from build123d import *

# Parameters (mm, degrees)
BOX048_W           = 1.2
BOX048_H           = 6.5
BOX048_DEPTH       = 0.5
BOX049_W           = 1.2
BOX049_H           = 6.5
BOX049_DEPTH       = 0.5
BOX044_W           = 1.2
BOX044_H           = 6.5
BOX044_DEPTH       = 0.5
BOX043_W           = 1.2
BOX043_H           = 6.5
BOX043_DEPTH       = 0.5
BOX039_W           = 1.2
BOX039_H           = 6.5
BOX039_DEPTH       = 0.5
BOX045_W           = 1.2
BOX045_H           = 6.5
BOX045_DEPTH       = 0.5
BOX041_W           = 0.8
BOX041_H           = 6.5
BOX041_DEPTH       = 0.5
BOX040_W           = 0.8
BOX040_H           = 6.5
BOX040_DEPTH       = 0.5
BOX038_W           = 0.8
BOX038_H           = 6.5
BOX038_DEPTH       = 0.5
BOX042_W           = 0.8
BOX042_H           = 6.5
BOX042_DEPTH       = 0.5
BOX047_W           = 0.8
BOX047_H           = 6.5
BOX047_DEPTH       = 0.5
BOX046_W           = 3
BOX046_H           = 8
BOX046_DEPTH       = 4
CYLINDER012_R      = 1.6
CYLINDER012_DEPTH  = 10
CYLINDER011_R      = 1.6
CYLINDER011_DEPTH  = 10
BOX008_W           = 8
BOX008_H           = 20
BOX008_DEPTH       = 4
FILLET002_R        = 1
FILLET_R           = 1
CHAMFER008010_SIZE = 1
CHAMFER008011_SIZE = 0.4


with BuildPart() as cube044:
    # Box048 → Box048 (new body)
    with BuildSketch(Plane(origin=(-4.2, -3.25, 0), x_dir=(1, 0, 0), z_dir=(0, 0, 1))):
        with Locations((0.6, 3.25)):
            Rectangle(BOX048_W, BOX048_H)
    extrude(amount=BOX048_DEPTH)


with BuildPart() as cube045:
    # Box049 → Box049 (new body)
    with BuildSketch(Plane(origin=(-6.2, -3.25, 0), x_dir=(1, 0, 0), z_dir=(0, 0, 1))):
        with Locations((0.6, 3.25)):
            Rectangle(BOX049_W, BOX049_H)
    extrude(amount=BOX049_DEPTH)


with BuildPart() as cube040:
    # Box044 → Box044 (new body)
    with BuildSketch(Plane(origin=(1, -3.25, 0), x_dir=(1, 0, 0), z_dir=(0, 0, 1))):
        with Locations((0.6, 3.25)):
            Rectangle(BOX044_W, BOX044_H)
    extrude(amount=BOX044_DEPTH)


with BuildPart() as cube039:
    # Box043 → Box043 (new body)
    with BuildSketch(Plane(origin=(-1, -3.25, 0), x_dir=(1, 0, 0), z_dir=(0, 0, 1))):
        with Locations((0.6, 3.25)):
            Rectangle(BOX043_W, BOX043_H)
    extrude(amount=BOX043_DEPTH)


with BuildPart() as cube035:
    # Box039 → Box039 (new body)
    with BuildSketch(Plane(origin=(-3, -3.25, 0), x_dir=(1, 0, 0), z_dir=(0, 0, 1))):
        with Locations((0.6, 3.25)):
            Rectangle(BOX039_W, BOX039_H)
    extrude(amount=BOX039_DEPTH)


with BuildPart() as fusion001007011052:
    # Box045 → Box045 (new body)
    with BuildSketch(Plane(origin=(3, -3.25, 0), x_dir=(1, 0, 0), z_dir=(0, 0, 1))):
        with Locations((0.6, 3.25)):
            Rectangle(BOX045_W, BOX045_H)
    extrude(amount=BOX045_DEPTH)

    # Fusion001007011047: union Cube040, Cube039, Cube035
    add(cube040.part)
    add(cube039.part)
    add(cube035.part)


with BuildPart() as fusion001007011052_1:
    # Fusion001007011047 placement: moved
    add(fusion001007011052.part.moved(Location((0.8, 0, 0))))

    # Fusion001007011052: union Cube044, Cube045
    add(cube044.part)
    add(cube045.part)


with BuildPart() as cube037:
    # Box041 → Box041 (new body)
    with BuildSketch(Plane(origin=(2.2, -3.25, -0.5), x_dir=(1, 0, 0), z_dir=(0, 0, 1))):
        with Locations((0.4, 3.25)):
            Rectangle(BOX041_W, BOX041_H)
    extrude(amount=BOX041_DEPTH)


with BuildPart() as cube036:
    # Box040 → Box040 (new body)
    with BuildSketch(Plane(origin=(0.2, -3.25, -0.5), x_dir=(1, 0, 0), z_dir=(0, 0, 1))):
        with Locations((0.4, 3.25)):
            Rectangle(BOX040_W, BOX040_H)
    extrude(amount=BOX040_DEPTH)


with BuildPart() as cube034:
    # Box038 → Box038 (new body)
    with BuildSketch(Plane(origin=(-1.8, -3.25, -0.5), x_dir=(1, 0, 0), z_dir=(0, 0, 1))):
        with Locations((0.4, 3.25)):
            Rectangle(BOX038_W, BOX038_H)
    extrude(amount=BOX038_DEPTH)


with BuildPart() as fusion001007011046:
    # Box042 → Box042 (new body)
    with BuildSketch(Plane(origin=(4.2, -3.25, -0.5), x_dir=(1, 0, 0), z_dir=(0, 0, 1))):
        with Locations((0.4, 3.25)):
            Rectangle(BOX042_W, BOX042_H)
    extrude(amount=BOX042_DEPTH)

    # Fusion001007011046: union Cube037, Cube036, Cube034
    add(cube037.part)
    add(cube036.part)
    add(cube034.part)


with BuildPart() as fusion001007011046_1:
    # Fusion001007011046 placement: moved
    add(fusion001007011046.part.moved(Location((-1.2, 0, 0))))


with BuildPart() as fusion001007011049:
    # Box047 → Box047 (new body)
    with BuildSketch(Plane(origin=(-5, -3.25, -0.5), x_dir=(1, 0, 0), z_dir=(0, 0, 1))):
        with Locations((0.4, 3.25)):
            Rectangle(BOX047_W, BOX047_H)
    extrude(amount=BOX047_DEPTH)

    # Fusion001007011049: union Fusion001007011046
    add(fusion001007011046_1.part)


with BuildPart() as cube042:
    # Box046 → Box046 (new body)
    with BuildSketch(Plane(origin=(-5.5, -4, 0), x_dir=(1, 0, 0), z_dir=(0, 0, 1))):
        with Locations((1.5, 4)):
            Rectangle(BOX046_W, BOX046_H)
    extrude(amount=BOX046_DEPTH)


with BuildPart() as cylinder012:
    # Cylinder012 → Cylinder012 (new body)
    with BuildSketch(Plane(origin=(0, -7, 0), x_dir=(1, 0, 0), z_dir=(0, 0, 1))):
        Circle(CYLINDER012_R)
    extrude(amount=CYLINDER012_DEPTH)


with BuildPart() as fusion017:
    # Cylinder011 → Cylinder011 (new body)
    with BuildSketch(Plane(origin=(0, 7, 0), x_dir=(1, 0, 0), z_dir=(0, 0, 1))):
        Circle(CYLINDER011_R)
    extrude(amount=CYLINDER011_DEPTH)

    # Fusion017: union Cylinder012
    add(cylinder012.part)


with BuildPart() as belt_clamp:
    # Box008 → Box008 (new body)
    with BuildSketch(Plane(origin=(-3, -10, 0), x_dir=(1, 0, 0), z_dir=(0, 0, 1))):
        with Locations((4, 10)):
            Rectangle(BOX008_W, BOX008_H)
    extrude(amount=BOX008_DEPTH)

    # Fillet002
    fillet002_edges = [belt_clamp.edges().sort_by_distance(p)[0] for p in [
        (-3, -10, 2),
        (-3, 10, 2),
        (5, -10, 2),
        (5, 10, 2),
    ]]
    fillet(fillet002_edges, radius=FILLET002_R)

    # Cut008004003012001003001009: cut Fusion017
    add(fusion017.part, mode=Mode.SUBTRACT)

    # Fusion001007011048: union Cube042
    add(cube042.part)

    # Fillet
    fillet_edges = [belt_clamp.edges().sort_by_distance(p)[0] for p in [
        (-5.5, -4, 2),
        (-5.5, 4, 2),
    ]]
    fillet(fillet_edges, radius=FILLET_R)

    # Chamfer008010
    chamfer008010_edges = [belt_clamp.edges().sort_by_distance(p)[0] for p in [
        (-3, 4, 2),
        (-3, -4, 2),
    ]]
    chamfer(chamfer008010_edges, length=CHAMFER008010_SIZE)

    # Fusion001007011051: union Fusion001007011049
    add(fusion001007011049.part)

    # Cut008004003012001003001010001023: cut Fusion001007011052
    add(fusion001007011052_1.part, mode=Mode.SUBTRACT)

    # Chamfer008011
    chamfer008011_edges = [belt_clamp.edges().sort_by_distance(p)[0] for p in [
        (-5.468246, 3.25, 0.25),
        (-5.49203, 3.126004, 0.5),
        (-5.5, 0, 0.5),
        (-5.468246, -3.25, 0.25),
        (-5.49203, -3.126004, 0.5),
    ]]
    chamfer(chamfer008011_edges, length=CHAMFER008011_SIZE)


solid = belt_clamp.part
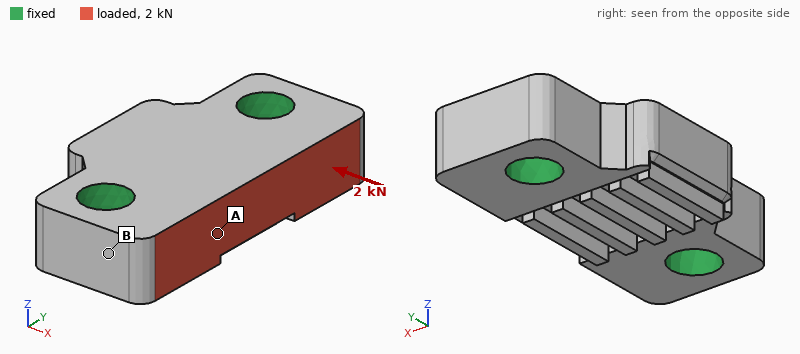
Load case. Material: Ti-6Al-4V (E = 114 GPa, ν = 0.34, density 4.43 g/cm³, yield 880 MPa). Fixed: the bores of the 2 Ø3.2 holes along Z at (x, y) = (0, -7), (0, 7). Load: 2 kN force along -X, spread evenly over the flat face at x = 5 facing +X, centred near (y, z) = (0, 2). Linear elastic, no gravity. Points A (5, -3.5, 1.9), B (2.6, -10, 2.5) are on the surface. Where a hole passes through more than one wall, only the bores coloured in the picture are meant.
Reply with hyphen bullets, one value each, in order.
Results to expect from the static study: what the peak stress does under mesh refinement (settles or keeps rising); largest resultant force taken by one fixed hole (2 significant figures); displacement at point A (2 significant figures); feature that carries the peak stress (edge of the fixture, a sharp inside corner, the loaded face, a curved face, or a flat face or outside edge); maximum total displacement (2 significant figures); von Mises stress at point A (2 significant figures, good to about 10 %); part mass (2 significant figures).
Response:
- keeps rising
- 1.0 kN
- 2.1 µm
- edge of the fixture
- 2.9 µm
- 25 MPa
- 2.9 g
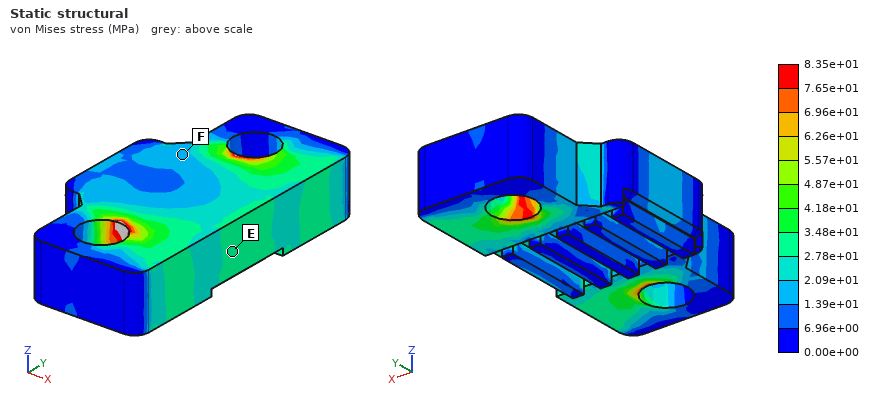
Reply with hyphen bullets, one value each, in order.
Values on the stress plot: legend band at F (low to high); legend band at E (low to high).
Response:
- 1.39e+01 to 2.09e+01 MPa
- 2.78e+01 to 3.48e+01 MPa
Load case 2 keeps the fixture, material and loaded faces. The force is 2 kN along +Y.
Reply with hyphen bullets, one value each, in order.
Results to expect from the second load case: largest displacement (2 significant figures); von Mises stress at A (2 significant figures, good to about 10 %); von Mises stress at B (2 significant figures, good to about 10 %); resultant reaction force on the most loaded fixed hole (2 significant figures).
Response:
- 4.0 µm
- 52 MPa
- 40 MPa
- 1.1 kN
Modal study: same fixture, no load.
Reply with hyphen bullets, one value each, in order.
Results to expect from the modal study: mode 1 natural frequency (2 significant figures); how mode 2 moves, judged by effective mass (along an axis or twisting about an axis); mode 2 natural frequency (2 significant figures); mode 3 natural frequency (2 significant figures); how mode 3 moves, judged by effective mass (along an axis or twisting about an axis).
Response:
- 66 kHz
- along Z
- 79 kHz
- 96 kHz
- along X
